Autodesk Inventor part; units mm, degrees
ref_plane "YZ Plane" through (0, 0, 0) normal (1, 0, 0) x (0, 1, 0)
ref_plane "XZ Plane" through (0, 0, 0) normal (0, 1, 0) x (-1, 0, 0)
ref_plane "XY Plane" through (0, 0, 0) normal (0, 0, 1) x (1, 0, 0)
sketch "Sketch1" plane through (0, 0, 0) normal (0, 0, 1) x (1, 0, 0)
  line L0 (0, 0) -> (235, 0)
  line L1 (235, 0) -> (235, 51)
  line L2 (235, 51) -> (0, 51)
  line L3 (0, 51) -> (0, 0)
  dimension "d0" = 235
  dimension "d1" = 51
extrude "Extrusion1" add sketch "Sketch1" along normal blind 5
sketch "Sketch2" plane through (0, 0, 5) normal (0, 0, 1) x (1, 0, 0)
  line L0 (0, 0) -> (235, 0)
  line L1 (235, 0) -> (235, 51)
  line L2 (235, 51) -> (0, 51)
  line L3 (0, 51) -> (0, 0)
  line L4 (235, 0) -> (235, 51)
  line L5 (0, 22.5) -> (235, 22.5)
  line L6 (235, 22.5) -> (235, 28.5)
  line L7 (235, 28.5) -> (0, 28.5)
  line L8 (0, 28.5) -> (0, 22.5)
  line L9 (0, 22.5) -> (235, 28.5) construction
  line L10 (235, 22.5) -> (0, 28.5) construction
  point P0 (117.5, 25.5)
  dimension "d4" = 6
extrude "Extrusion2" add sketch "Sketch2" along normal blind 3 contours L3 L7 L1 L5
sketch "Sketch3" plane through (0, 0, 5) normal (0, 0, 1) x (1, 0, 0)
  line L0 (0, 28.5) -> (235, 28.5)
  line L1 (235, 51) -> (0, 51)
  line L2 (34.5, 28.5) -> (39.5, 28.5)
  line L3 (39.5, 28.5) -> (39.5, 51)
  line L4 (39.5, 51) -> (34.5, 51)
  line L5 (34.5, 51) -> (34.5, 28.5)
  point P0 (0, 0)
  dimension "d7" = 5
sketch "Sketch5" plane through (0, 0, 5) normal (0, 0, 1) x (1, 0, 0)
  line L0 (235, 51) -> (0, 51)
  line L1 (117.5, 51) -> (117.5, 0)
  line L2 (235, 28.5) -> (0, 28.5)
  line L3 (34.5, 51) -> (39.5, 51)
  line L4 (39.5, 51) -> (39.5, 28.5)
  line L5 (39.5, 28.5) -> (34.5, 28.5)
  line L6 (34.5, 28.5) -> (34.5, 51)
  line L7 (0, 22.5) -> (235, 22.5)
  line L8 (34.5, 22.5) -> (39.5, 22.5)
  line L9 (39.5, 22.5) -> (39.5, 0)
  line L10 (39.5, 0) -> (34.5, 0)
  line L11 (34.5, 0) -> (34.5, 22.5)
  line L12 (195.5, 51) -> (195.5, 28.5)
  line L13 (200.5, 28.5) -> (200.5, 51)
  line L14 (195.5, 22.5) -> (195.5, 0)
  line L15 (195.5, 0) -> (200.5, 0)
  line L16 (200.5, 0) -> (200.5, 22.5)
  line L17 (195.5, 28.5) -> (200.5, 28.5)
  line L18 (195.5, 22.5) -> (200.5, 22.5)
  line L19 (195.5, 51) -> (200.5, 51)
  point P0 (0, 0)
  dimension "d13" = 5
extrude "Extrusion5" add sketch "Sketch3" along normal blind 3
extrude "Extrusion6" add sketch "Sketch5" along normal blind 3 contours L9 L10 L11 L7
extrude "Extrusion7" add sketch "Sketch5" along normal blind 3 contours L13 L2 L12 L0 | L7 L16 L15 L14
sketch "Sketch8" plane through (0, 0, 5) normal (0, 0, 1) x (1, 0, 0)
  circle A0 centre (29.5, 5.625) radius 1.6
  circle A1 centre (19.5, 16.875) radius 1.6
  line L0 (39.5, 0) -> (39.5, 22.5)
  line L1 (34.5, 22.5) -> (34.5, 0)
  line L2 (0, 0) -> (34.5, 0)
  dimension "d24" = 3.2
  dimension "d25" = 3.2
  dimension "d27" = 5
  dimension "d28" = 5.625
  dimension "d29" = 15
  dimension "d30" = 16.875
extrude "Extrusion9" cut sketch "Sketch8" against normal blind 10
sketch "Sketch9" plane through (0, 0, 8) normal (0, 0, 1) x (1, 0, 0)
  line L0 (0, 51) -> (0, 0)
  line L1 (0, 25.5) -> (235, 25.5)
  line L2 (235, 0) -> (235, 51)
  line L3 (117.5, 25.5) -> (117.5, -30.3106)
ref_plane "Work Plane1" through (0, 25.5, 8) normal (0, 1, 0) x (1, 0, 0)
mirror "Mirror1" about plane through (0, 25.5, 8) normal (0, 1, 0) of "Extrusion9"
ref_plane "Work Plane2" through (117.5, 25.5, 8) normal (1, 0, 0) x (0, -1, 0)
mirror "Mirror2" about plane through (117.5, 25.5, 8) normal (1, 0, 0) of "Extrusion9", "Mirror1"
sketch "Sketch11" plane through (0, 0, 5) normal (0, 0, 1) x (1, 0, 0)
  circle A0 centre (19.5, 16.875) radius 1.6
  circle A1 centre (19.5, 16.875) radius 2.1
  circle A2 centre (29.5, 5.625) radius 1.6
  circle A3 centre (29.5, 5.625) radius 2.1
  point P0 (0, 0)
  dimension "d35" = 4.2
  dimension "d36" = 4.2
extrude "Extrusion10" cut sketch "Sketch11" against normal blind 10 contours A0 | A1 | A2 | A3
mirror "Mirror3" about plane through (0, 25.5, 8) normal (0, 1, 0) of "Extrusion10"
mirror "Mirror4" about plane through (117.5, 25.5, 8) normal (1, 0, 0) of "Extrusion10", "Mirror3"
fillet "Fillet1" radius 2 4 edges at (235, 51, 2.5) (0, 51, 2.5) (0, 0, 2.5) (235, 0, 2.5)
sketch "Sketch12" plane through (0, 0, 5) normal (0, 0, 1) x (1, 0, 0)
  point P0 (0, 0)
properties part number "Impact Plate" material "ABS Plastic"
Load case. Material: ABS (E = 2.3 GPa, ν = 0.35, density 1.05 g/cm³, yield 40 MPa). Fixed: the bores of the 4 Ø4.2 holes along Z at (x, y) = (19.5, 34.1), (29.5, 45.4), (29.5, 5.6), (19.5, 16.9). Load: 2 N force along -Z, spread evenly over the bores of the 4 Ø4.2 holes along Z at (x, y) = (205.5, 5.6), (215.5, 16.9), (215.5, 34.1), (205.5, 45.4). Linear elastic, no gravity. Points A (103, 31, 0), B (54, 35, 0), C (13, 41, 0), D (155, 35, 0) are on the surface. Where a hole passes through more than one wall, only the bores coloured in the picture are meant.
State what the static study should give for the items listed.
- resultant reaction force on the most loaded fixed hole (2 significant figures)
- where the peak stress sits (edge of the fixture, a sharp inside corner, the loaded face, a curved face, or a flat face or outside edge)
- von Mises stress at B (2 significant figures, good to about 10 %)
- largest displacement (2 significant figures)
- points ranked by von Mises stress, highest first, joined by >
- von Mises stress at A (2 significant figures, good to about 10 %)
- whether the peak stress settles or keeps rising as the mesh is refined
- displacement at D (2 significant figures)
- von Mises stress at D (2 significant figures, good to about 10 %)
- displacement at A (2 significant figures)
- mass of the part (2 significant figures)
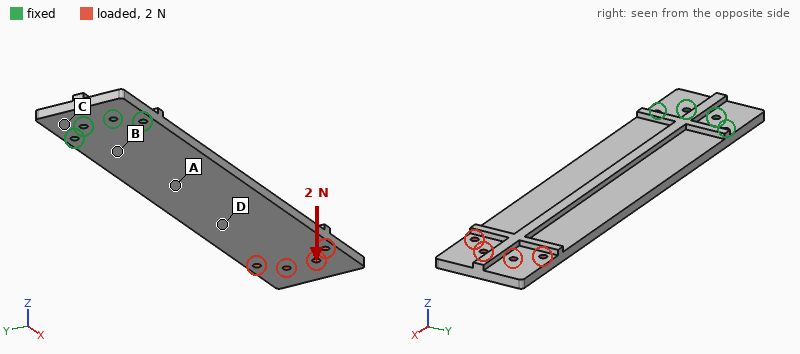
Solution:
8.1 N
edge of the fixture
1.0 MPa
2.6 mm
B > A > D > C
0.73 MPa
keeps rising
1.2 mm
0.38 MPa
0.48 mm
68 g
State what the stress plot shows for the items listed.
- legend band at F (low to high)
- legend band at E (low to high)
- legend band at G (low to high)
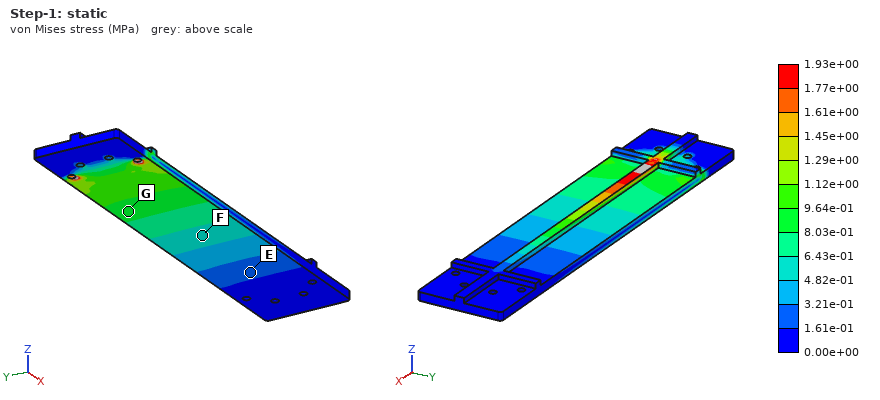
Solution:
4.82e-01 to 6.43e-01 MPa
1.61e-01 to 3.21e-01 MPa
8.03e-01 to 9.64e-01 MPa
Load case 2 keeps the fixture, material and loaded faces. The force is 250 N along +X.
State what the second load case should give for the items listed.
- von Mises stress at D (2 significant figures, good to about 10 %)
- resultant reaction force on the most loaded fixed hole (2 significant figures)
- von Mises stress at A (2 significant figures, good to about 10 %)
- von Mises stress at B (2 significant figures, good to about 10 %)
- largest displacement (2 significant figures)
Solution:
1.1 MPa
79 N
1.1 MPa
1.1 MPa
0.73 mm
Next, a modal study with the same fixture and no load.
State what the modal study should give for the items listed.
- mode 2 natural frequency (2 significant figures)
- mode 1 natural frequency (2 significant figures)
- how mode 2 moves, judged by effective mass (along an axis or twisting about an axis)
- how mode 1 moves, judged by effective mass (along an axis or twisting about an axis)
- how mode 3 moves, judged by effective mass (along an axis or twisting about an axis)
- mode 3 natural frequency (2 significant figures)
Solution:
210 Hz
33 Hz
along Z
along Z
twisting about X
240 Hz
